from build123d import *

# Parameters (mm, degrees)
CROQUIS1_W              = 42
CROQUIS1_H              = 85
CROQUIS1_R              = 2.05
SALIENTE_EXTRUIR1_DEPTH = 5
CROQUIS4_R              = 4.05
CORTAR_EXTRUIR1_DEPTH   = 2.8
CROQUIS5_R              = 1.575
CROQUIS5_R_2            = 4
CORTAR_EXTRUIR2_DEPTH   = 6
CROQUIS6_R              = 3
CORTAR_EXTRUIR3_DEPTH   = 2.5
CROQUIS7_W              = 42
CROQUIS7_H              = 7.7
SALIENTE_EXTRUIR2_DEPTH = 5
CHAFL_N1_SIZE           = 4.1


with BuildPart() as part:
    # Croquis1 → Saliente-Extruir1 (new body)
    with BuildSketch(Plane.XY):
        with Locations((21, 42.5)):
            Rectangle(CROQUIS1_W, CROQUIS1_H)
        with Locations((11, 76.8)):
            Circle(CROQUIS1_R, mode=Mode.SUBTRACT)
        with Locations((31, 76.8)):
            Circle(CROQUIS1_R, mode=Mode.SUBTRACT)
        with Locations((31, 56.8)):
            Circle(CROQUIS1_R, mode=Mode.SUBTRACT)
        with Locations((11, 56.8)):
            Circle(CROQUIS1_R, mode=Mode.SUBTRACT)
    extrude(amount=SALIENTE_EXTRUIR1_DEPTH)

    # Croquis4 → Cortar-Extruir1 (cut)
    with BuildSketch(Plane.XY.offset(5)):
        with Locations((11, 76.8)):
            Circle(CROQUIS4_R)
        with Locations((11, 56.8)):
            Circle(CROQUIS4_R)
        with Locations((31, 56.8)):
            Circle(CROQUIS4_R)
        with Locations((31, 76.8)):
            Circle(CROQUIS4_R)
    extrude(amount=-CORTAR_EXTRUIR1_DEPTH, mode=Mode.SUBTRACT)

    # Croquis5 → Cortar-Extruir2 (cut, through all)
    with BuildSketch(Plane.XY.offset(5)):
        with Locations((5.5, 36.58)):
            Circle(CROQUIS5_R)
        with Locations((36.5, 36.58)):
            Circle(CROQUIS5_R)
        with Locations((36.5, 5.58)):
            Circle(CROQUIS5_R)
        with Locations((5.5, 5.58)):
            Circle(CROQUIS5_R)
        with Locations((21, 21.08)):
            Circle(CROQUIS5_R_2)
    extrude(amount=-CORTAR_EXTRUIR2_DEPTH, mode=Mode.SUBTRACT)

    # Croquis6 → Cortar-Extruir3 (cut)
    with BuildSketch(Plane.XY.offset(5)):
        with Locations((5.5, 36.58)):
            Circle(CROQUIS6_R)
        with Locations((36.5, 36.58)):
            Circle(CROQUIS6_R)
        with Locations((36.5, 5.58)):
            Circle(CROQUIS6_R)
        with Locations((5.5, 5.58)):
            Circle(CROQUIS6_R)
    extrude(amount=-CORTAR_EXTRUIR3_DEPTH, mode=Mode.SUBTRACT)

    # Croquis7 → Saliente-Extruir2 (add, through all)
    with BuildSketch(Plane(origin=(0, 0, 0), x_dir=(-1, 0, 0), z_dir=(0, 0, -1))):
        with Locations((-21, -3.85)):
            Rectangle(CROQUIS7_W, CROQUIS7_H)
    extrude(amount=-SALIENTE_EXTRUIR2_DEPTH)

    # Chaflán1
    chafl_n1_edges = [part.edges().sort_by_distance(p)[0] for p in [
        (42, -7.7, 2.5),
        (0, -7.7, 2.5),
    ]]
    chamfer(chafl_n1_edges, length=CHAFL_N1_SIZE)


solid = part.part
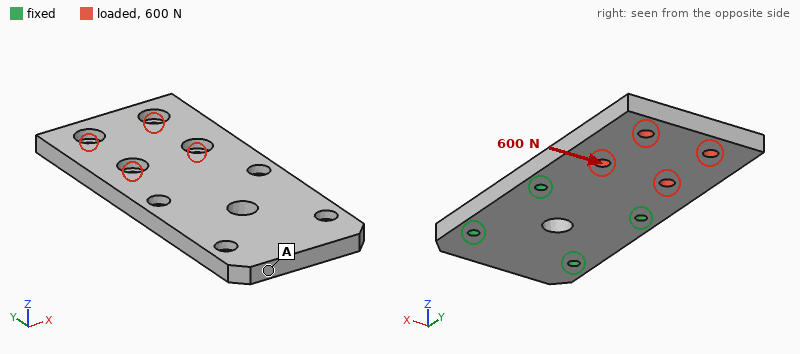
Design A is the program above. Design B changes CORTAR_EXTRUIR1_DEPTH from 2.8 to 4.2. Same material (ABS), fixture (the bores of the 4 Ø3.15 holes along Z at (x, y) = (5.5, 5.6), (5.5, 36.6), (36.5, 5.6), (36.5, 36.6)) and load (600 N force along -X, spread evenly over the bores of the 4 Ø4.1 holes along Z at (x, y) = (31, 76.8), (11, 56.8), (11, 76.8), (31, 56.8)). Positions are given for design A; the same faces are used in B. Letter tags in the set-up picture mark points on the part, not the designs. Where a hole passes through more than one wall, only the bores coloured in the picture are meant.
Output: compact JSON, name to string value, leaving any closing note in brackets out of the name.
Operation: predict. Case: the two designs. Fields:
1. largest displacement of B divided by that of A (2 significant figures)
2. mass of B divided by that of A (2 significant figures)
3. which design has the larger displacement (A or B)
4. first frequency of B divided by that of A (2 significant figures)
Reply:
{"largest displacement of B divided by that of A": "1.3", "mass of B divided by that of A": "0.99", "which design has the larger displacement": "B", "first frequency of B divided by that of A": "1.0"}
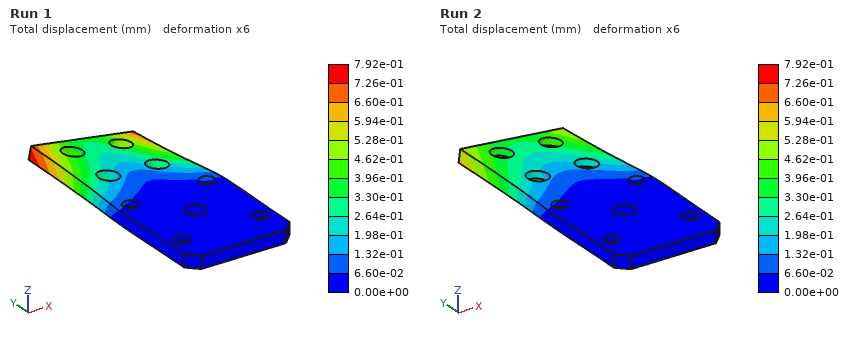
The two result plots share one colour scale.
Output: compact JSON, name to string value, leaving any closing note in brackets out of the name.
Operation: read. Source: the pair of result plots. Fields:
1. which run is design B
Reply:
{"which run is design B": "Run 1"}
